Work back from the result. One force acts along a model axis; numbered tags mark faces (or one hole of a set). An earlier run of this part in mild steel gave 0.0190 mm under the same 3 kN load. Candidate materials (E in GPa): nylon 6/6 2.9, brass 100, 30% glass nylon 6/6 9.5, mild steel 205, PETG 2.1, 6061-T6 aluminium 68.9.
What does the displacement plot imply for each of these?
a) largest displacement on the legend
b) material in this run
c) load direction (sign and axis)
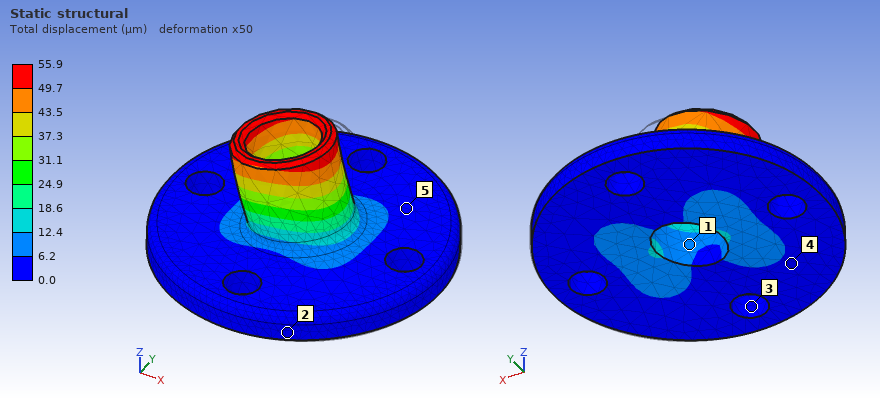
55.9 µm
6061-T6 aluminium
-X
